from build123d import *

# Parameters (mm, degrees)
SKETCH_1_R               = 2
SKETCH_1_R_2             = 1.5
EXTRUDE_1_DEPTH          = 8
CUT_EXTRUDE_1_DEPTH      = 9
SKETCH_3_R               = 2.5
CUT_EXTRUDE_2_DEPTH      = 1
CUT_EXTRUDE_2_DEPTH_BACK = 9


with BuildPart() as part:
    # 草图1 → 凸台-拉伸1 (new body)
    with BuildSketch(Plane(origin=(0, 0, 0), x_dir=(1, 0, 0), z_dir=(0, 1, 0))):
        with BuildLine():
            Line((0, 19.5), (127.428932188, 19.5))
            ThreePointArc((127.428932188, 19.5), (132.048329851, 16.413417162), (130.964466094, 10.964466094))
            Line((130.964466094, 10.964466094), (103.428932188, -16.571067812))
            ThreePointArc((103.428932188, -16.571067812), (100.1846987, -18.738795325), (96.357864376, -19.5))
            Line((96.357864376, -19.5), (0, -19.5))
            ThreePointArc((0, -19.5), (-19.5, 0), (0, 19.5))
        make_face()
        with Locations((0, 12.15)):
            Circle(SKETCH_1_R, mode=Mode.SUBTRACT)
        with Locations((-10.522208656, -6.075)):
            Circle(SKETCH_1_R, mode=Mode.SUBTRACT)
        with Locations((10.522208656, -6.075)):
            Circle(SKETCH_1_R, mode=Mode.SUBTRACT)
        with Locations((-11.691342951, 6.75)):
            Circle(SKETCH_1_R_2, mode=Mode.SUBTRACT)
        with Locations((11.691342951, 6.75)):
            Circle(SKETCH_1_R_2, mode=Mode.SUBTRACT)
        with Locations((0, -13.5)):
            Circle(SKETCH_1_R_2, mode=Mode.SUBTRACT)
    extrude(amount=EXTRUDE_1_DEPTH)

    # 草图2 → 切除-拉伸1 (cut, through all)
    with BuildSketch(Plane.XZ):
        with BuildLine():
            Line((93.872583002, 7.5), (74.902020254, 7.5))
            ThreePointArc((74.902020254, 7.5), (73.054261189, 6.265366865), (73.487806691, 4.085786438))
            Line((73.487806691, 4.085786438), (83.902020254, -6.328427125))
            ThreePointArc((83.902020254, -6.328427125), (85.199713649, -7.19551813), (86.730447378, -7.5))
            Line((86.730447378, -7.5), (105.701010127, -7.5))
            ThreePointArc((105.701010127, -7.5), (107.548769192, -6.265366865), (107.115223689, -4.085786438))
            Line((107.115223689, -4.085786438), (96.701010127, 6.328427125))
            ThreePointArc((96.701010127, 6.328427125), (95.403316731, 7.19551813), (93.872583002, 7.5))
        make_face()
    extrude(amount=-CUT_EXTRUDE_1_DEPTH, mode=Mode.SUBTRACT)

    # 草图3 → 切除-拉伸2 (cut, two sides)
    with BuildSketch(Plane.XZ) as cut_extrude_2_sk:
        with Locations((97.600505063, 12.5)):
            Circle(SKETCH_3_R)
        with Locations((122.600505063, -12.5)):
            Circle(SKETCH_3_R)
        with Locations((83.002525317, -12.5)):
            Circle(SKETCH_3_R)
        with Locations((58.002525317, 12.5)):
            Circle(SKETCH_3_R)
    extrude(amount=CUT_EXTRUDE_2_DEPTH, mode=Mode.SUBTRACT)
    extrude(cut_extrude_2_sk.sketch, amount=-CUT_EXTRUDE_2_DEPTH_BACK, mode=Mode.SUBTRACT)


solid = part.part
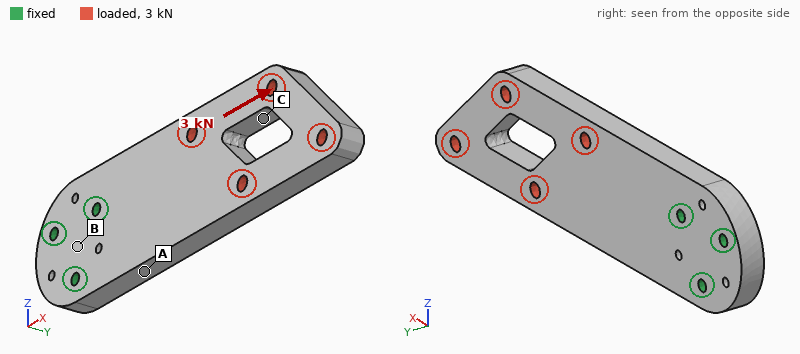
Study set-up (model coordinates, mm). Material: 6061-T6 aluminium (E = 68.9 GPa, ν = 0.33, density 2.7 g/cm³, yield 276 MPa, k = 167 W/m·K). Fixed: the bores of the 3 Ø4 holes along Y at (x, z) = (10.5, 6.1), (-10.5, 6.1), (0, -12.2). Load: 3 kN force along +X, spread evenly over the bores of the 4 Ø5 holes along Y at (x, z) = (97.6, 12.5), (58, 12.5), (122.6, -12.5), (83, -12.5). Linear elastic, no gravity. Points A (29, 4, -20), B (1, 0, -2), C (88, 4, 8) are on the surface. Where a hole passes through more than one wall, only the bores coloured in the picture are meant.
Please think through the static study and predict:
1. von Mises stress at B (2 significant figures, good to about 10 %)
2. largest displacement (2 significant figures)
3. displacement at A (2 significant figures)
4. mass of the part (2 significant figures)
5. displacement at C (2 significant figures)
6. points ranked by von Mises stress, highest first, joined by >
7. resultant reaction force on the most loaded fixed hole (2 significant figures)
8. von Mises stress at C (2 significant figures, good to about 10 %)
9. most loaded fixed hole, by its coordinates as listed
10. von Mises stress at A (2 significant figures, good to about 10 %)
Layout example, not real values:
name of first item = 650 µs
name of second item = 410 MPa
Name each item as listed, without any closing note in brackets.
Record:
von Mises stress at B = 3.2 MPa
largest displacement = 22 µm
displacement at A = 4.6 µm
mass of the part = 100 g
displacement at C = 12 µm
points ranked by von Mises stress, highest first, joined by > = C > A > B
resultant reaction force on the most loaded fixed hole = 1.6 kN
von Mises stress at C = 13 MPa
most loaded fixed hole, by its coordinates as listed = (10.5, 6.1)
von Mises stress at A = 9.2 MPa
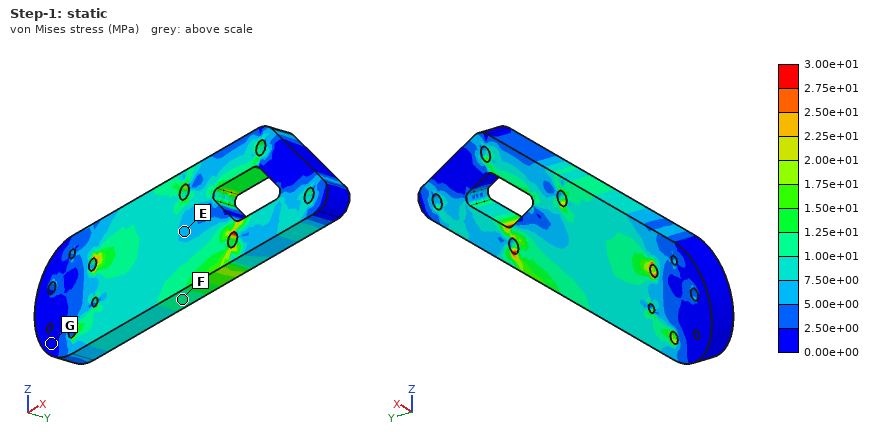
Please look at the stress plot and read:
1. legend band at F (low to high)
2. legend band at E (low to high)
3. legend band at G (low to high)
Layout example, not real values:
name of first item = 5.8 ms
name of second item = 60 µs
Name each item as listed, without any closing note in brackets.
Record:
legend band at F = 1.00e+01 to 1.25e+01 MPa
legend band at E = 5.00e+00 to 7.50e+00 MPa
legend band at G = 0.00e+00 to 2.50e+00 MPa
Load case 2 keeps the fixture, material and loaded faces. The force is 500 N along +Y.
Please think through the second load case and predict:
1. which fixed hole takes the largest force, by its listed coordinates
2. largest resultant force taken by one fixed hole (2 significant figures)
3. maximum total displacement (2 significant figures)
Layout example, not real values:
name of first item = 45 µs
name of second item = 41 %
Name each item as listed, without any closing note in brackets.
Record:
which fixed hole takes the largest force, by its listed coordinates = (10.5, 6.1)
largest resultant force taken by one fixed hole = 1.4 kN
maximum total displacement = 1.6 mm
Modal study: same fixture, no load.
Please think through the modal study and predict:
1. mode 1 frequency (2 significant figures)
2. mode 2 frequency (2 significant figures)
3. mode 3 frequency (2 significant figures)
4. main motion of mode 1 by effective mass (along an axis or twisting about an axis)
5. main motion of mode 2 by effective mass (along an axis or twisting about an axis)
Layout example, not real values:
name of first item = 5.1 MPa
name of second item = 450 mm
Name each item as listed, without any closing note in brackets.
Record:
mode 1 frequency = 560 Hz
mode 2 frequency = 2200 Hz
mode 3 frequency = 2600 Hz
main motion of mode 1 by effective mass = along Y
main motion of mode 2 by effective mass = along Z
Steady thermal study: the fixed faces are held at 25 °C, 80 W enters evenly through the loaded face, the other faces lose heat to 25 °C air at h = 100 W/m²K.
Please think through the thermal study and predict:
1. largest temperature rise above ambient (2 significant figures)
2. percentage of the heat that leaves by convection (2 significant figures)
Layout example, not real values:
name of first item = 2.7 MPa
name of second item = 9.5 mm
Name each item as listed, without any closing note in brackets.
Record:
largest temperature rise above ambient = 80 K
percentage of the heat that leaves by convection = 55 %
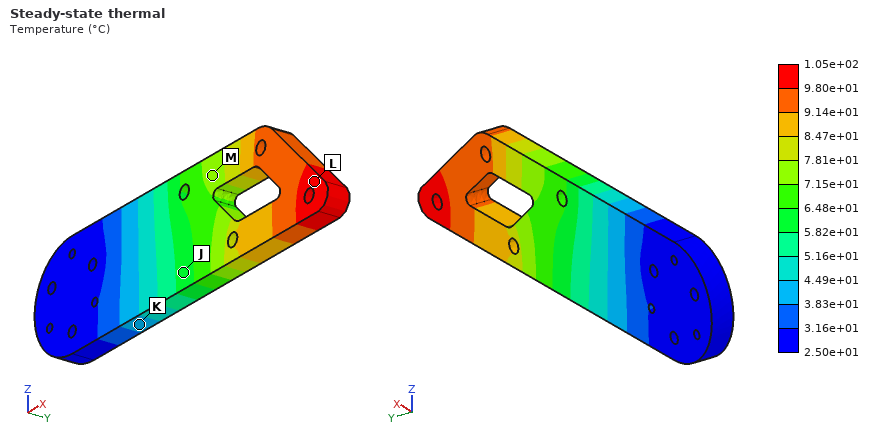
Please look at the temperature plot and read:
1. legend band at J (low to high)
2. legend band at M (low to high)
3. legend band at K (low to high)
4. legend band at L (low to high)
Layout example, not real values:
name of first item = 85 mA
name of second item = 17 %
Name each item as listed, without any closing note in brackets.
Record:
legend band at J = 5.82e+01 to 6.48e+01 °C
legend band at M = 7.15e+01 to 7.81e+01 °C
legend band at K = 3.83e+01 to 4.49e+01 °C
legend band at L = 9.80e+01 to 1.05e+02 °C
